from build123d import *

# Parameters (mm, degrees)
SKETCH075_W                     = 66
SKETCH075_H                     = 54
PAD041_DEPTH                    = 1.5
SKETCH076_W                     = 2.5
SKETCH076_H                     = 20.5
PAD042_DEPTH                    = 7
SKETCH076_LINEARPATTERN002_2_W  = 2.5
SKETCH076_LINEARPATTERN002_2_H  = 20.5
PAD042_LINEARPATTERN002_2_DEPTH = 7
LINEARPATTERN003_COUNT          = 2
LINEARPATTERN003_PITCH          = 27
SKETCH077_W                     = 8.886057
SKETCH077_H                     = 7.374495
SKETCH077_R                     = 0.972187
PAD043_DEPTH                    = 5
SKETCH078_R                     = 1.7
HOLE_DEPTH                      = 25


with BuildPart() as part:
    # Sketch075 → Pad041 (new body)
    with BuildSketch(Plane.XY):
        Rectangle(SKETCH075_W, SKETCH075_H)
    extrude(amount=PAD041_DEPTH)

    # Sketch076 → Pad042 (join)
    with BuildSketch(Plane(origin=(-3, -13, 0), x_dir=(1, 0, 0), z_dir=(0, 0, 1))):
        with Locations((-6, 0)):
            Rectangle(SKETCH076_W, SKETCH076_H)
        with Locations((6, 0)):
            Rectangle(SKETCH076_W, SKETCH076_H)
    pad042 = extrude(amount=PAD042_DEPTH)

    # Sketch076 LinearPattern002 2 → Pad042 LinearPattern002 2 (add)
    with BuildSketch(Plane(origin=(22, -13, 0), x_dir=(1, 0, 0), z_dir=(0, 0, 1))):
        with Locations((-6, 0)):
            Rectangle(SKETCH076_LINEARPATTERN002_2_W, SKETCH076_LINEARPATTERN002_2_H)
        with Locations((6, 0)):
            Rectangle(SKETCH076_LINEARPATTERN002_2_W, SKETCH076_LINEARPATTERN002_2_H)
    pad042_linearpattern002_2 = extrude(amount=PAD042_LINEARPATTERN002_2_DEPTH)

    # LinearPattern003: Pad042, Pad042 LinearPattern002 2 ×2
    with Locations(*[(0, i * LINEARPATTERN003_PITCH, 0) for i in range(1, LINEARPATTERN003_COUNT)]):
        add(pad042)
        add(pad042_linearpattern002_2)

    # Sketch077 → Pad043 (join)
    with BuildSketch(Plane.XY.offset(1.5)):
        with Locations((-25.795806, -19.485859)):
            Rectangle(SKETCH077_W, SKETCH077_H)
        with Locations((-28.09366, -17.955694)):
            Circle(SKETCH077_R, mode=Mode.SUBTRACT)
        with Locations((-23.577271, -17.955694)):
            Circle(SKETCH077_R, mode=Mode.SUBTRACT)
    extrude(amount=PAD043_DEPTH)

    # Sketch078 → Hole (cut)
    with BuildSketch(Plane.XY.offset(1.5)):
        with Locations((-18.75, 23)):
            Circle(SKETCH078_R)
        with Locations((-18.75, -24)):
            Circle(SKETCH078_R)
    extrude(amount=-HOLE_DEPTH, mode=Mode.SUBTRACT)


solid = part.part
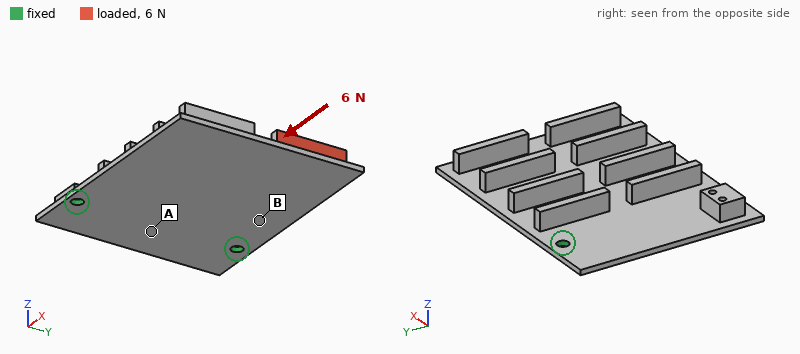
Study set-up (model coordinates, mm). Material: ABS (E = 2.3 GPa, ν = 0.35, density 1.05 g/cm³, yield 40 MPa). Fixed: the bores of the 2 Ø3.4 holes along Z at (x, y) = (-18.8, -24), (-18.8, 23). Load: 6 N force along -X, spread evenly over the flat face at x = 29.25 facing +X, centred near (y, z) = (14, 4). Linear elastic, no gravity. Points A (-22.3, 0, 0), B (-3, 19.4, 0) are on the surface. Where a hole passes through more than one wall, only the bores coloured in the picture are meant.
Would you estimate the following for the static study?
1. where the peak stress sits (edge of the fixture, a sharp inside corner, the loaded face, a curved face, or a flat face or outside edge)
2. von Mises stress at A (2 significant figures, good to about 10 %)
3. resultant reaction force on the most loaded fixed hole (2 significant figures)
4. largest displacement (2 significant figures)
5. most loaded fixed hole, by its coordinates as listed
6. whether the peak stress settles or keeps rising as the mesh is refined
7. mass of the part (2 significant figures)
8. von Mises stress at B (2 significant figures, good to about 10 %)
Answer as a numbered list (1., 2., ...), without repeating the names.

1. edge of the fixture
2. 0.30 MPa
3. 4.8 N
4. 0.83 mm
5. (-18.8, 23)
6. keeps rising
7. 8.3 g
8. 0.81 MPa
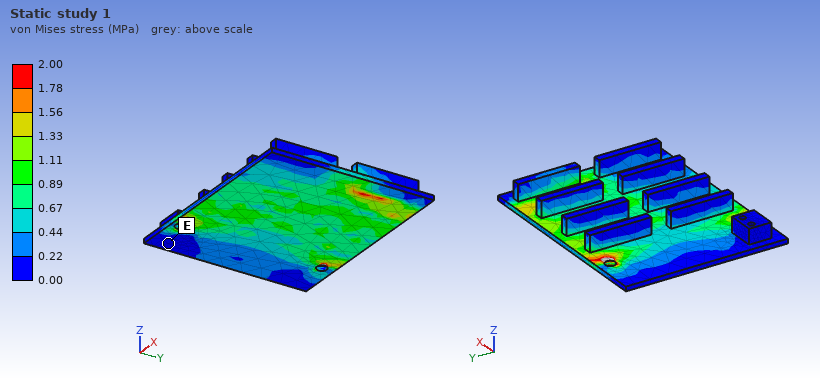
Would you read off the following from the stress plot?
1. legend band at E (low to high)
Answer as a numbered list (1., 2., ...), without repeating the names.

1. 0.00 to 0.22 MPa
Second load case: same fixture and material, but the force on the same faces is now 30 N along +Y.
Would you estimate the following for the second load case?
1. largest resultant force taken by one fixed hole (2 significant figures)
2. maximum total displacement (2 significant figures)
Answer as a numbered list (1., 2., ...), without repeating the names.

1. 34 N
2. 1.0 mm
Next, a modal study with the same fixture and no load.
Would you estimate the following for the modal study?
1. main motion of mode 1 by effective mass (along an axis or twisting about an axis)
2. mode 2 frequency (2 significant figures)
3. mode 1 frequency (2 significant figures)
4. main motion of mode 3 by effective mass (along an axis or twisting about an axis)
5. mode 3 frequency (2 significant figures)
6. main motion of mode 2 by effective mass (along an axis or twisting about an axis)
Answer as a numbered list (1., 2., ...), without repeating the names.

1. along Z
2. 340 Hz
3. 100 Hz
4. along Z
5. 630 Hz
6. twisting about X
